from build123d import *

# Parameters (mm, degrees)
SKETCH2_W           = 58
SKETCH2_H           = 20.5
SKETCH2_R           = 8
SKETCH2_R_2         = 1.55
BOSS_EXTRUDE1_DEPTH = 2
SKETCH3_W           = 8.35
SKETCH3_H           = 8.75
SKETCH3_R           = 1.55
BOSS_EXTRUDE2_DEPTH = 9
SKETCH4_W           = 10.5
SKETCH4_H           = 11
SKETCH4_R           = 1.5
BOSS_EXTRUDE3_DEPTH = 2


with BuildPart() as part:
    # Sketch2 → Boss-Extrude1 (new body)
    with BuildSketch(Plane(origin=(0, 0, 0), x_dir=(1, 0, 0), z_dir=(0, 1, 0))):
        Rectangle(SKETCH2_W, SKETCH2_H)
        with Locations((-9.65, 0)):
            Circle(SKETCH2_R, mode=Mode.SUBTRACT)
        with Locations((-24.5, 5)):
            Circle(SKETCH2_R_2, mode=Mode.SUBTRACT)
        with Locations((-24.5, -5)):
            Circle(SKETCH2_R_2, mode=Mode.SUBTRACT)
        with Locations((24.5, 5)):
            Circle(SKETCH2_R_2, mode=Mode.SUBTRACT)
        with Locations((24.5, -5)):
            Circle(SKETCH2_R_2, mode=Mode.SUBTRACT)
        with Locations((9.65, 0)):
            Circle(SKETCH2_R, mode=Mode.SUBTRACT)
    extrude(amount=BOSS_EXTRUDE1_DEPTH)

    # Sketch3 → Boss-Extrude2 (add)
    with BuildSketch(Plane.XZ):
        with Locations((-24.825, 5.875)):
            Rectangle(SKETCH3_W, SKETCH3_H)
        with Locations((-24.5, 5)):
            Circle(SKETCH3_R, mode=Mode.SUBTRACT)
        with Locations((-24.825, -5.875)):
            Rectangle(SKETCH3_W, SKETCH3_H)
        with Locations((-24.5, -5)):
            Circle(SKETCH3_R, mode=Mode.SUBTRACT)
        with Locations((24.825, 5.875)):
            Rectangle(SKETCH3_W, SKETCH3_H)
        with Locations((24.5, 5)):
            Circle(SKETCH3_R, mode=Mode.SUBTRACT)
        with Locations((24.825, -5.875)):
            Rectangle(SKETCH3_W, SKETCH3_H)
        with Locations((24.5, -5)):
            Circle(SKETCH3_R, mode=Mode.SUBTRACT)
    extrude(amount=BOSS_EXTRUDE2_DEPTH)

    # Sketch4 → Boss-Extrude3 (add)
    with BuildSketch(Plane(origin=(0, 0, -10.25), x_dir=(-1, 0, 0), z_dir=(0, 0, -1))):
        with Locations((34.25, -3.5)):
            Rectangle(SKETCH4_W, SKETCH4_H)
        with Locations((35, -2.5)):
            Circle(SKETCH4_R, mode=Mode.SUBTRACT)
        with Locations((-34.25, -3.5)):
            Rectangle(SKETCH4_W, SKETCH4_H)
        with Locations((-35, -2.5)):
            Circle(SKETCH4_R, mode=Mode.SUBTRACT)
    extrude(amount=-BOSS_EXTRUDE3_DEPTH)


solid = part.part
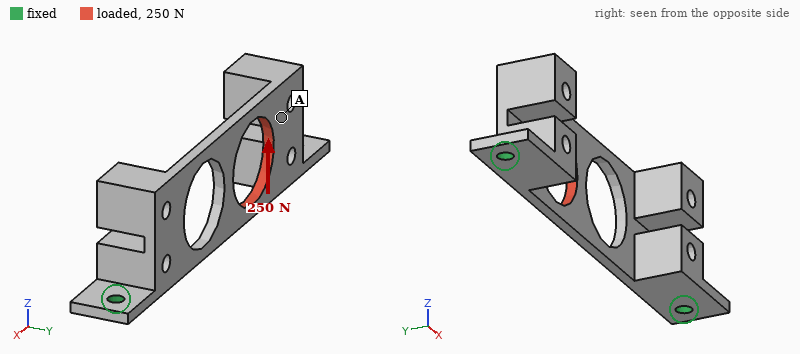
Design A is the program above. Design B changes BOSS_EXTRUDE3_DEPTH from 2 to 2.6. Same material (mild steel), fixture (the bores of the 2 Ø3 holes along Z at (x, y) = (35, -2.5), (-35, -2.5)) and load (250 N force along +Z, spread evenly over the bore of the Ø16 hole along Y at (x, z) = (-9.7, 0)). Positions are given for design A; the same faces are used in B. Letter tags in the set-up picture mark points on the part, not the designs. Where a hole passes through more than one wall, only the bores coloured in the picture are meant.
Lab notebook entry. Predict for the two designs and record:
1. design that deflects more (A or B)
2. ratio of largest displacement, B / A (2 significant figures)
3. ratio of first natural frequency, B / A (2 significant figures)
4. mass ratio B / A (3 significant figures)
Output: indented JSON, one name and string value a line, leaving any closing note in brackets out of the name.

{
  "design that deflects more": "A",
  "ratio of largest displacement, B / A": "0.69",
  "ratio of first natural frequency, B / A": "1.2",
  "mass ratio B / A": "1.03"
}
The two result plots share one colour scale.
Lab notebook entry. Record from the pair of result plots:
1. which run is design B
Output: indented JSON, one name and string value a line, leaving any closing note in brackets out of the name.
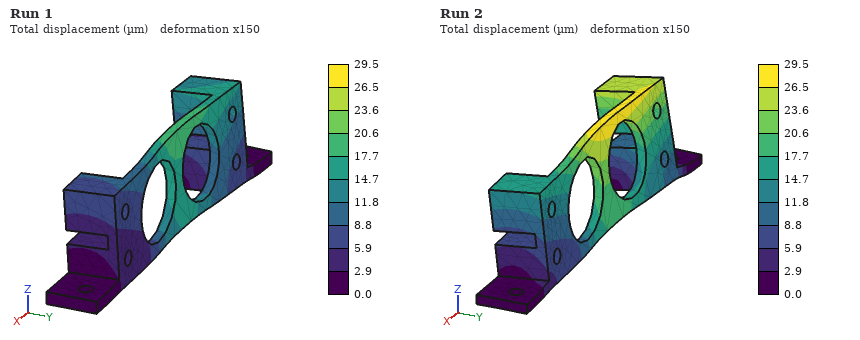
{
  "which run is design B": "Run 1"
}
